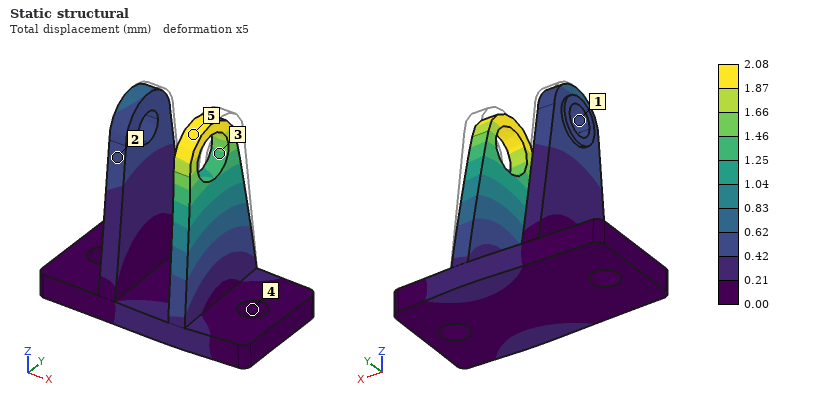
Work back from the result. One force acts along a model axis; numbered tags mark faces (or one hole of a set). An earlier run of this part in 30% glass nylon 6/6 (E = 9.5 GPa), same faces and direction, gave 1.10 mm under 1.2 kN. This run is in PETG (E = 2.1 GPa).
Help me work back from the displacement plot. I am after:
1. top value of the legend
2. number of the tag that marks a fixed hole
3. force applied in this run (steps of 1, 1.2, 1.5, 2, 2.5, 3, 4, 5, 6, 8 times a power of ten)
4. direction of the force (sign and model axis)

2.08 mm
4
500 N
-Y
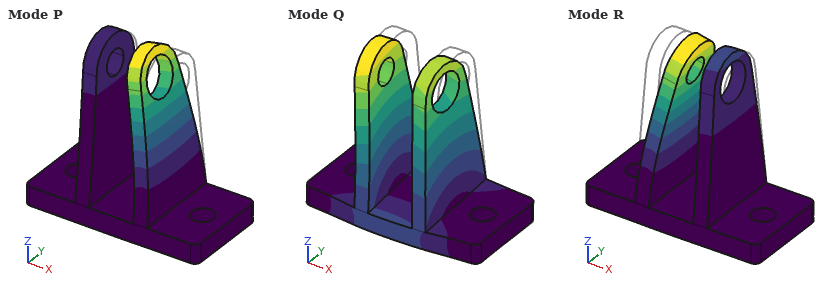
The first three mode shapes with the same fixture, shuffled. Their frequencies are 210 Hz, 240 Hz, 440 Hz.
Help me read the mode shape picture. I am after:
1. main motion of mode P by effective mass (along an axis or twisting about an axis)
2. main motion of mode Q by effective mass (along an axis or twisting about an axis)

along X
along Y
